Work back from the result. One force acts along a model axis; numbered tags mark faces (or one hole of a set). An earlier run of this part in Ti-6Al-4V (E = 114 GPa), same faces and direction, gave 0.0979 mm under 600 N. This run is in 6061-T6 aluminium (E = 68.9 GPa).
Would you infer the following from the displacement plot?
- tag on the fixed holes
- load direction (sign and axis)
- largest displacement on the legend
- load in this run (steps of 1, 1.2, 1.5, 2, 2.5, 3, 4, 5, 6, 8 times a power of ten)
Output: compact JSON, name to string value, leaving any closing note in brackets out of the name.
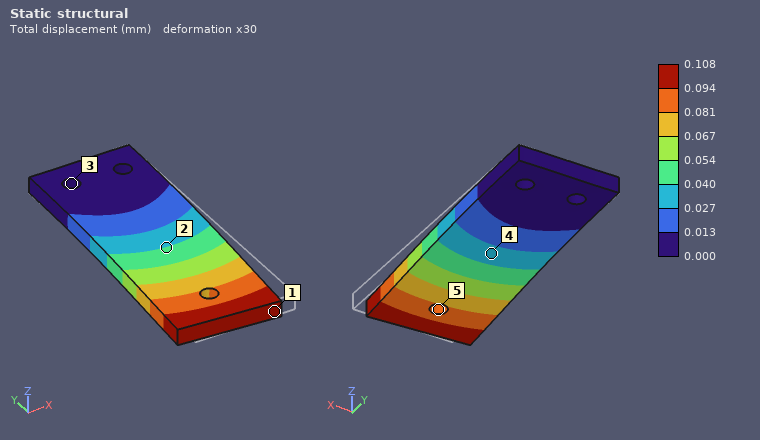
{"tag on the fixed holes": "3", "load direction": "-X", "largest displacement on the legend": "0.108 mm", "load in this run": "400 N"}
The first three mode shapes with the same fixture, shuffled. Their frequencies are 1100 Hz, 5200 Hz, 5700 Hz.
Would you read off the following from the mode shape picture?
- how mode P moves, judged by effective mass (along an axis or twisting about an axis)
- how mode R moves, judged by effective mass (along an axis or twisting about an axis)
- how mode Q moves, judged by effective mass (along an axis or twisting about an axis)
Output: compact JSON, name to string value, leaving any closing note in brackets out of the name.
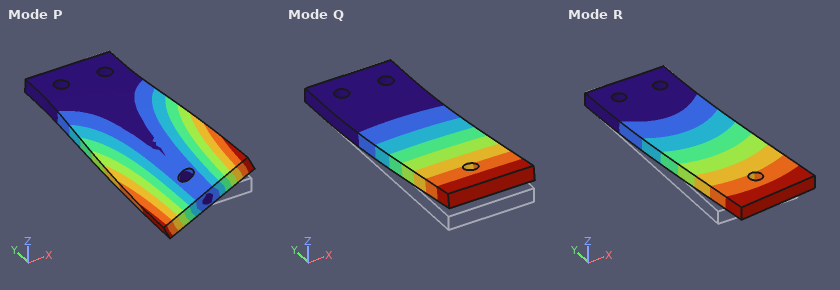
{"how mode P moves, judged by effective mass": "twisting about Y", "how mode R moves, judged by effective mass": "along X", "how mode Q moves, judged by effective mass": "along Z"}
